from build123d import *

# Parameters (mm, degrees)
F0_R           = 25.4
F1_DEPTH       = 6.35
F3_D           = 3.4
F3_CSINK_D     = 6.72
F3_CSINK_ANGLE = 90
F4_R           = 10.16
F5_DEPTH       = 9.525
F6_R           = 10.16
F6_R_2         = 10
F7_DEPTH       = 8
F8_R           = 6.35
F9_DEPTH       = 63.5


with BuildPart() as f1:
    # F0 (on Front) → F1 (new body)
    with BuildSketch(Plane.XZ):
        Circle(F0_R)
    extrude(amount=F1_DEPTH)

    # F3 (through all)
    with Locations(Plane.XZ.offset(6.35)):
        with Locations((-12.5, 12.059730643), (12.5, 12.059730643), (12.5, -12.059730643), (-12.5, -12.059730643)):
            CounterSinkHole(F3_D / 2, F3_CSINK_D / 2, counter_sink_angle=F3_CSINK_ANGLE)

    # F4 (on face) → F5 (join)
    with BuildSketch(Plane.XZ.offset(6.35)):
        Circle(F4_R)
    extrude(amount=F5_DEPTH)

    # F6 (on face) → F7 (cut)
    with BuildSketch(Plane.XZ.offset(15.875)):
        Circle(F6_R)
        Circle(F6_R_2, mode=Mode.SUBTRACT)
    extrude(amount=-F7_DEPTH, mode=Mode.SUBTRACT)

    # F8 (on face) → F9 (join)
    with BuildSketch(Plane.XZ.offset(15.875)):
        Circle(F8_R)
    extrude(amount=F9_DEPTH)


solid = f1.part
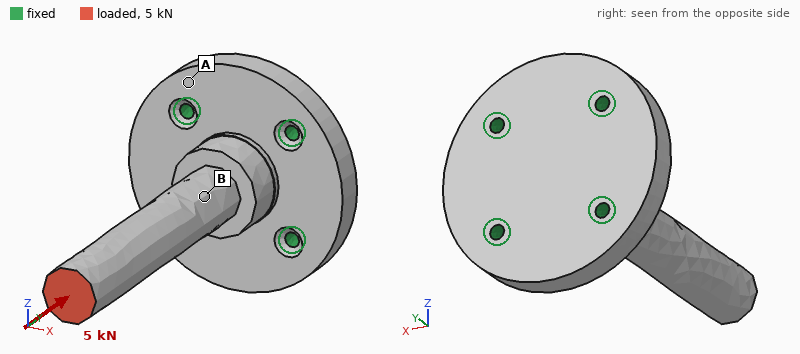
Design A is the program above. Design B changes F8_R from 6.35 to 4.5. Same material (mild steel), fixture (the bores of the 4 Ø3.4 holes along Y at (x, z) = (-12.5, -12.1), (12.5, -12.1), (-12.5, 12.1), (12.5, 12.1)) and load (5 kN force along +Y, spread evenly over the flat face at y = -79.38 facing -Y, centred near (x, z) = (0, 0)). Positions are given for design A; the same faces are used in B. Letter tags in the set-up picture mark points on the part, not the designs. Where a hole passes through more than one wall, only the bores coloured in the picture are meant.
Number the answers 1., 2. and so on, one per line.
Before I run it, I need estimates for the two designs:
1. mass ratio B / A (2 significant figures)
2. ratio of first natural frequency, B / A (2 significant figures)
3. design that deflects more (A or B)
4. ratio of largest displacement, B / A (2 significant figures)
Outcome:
1. 0.83
2. 0.78
3. B
4. 1.7
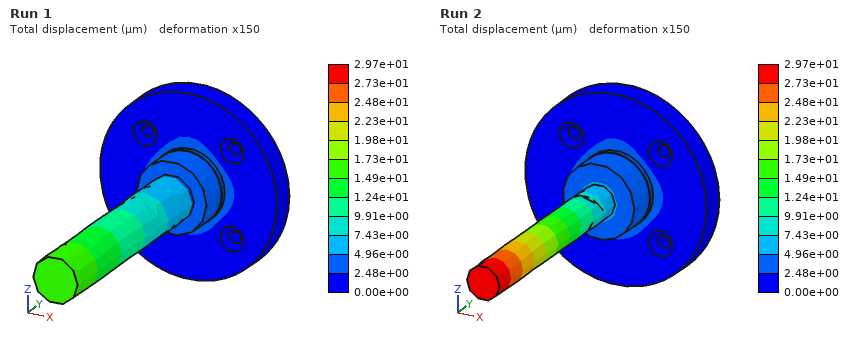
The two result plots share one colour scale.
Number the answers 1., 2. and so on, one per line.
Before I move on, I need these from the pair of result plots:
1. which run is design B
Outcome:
1. Run 2
